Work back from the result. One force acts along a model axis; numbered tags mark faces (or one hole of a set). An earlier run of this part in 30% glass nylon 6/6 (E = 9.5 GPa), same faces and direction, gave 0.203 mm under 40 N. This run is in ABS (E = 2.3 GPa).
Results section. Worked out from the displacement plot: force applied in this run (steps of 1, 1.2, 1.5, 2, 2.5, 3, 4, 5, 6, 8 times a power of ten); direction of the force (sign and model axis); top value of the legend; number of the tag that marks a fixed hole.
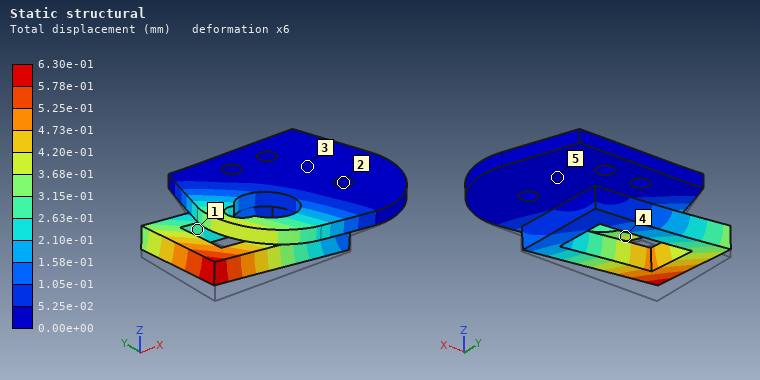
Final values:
30 N
+Z
6.30e-01 mm
2
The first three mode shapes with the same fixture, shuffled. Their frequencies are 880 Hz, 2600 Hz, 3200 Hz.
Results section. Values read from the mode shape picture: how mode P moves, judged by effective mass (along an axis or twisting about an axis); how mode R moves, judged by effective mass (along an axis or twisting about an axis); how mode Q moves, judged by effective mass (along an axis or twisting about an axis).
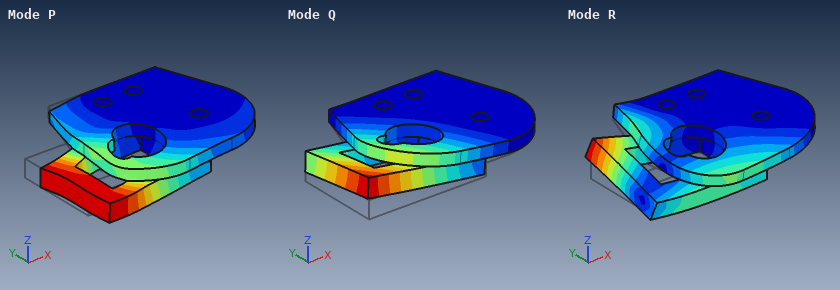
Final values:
along Y
twisting about X
along Z
